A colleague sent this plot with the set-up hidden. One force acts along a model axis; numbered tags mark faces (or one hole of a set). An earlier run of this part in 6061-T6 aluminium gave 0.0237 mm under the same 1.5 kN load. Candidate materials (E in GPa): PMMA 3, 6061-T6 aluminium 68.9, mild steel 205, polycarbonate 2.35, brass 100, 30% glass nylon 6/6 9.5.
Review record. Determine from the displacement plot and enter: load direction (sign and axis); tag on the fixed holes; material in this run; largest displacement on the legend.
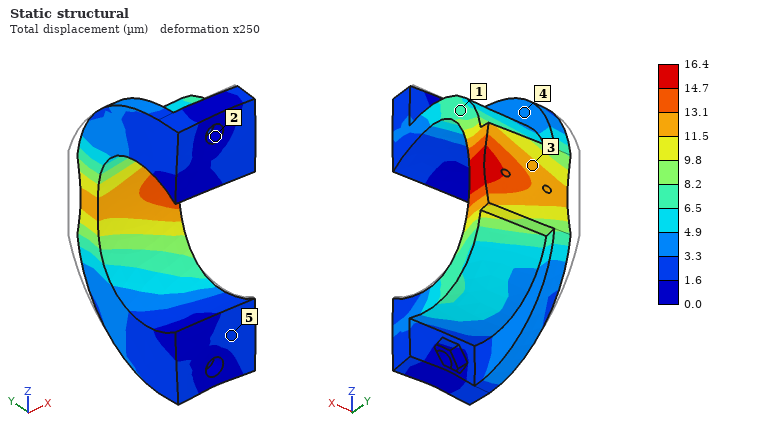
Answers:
-Y
2
brass
16.4 µm
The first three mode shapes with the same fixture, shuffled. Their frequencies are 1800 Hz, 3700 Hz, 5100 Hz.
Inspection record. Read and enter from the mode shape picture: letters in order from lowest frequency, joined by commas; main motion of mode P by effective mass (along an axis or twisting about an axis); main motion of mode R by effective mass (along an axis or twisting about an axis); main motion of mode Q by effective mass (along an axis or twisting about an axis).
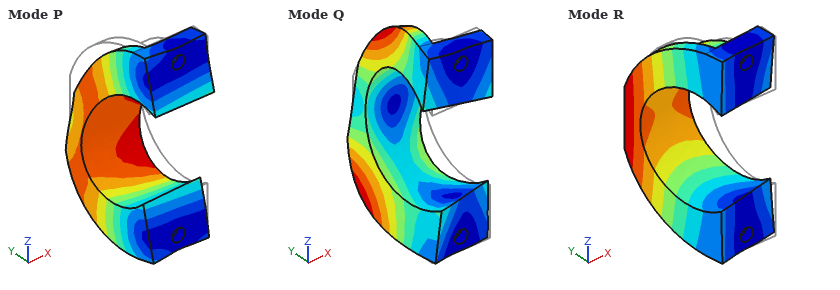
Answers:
R, P, Q
along Z
along X
twisting about Y
